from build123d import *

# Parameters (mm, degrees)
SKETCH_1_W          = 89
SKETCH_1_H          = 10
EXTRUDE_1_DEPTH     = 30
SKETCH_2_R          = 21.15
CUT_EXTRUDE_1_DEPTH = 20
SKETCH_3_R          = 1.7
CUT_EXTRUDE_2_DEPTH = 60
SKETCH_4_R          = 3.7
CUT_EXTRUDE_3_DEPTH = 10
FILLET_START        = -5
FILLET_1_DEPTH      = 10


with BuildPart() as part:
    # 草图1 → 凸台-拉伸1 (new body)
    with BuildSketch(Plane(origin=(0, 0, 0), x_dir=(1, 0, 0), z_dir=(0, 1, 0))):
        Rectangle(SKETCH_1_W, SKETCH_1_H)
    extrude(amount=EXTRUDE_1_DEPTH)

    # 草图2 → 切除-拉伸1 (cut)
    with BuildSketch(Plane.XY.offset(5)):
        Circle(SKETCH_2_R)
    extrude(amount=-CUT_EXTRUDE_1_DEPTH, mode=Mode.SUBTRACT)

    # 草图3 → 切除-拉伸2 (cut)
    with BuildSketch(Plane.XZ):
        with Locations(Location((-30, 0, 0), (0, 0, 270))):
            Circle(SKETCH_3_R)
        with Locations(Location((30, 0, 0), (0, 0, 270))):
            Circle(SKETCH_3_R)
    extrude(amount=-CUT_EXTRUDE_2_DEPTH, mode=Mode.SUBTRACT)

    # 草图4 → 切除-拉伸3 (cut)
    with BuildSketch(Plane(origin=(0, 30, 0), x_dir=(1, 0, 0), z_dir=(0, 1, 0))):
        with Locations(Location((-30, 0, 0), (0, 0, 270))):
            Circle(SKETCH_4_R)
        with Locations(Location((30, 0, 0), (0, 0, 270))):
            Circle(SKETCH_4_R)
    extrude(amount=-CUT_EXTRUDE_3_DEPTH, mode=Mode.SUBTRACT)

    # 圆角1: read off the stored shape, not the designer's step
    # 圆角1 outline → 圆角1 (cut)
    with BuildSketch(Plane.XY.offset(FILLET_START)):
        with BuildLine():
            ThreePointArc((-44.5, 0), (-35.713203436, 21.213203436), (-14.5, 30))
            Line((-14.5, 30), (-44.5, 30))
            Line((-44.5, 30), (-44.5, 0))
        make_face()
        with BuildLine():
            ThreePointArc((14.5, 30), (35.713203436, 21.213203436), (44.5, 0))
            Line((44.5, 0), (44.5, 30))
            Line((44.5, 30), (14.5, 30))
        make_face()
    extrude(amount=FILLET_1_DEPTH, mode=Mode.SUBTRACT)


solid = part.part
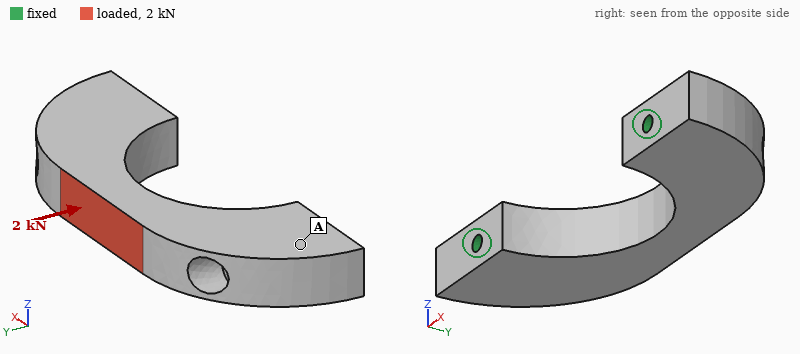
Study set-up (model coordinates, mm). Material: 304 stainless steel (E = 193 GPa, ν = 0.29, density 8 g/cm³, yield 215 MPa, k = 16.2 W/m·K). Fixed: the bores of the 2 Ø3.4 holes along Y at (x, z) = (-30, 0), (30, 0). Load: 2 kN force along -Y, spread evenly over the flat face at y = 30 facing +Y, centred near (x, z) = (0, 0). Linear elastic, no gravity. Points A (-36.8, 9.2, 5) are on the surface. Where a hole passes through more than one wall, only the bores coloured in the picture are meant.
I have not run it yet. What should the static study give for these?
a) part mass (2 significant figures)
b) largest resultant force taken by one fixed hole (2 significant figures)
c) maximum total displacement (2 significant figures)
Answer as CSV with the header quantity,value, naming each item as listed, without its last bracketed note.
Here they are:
quantity,value
part mass,120 g
largest resultant force taken by one fixed hole,1.4 kN
maximum total displacement,4.6 µm
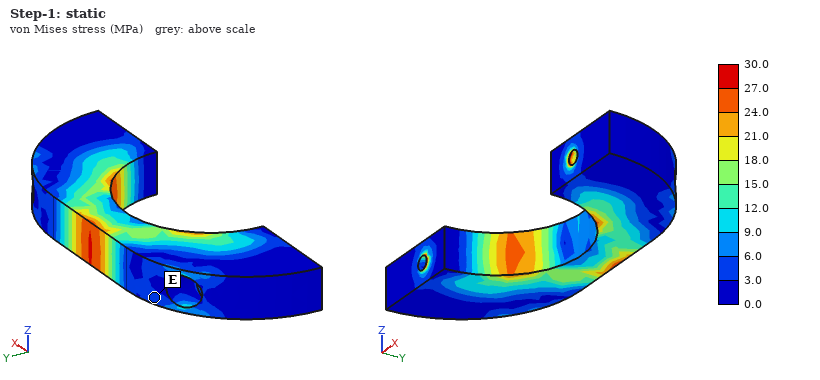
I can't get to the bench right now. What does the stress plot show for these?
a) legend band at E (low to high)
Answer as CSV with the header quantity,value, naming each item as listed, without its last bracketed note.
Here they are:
quantity,value
legend band at E,3.0 to 6.0 MPa
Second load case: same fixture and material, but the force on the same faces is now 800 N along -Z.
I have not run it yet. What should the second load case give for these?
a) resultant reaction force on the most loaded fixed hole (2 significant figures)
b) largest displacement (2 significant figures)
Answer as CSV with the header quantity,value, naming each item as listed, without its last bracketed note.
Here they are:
quantity,value
resultant reaction force on the most loaded fixed hole,400 N
largest displacement,11 µm
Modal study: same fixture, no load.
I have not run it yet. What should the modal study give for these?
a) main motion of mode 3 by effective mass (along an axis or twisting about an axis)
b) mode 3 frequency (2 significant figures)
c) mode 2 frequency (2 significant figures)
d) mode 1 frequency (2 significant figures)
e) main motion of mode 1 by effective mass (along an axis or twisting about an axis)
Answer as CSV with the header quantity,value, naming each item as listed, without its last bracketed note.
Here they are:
quantity,value
main motion of mode 3 by effective mass,along Y
mode 3 frequency,22 kHz
mode 2 frequency,21 kHz
mode 1 frequency,9700 Hz
main motion of mode 1 by effective mass,along Z
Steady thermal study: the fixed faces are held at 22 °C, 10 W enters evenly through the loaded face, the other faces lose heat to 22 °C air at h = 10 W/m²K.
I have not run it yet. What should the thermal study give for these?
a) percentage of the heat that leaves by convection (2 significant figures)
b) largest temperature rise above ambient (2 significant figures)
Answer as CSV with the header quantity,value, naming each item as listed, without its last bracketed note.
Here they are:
quantity,value
percentage of the heat that leaves by convection,7.7 %
largest temperature rise above ambient,61 K
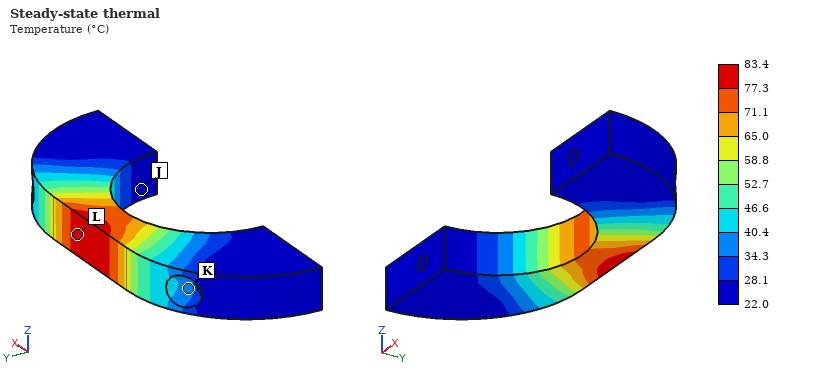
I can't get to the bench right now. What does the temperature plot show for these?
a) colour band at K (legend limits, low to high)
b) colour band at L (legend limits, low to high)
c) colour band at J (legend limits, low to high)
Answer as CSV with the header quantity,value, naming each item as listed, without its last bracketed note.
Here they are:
quantity,value
colour band at K,34.3 to 40.4 °C
colour band at L,77.3 to 83.4 °C
colour band at J,22.0 to 28.1 °C
